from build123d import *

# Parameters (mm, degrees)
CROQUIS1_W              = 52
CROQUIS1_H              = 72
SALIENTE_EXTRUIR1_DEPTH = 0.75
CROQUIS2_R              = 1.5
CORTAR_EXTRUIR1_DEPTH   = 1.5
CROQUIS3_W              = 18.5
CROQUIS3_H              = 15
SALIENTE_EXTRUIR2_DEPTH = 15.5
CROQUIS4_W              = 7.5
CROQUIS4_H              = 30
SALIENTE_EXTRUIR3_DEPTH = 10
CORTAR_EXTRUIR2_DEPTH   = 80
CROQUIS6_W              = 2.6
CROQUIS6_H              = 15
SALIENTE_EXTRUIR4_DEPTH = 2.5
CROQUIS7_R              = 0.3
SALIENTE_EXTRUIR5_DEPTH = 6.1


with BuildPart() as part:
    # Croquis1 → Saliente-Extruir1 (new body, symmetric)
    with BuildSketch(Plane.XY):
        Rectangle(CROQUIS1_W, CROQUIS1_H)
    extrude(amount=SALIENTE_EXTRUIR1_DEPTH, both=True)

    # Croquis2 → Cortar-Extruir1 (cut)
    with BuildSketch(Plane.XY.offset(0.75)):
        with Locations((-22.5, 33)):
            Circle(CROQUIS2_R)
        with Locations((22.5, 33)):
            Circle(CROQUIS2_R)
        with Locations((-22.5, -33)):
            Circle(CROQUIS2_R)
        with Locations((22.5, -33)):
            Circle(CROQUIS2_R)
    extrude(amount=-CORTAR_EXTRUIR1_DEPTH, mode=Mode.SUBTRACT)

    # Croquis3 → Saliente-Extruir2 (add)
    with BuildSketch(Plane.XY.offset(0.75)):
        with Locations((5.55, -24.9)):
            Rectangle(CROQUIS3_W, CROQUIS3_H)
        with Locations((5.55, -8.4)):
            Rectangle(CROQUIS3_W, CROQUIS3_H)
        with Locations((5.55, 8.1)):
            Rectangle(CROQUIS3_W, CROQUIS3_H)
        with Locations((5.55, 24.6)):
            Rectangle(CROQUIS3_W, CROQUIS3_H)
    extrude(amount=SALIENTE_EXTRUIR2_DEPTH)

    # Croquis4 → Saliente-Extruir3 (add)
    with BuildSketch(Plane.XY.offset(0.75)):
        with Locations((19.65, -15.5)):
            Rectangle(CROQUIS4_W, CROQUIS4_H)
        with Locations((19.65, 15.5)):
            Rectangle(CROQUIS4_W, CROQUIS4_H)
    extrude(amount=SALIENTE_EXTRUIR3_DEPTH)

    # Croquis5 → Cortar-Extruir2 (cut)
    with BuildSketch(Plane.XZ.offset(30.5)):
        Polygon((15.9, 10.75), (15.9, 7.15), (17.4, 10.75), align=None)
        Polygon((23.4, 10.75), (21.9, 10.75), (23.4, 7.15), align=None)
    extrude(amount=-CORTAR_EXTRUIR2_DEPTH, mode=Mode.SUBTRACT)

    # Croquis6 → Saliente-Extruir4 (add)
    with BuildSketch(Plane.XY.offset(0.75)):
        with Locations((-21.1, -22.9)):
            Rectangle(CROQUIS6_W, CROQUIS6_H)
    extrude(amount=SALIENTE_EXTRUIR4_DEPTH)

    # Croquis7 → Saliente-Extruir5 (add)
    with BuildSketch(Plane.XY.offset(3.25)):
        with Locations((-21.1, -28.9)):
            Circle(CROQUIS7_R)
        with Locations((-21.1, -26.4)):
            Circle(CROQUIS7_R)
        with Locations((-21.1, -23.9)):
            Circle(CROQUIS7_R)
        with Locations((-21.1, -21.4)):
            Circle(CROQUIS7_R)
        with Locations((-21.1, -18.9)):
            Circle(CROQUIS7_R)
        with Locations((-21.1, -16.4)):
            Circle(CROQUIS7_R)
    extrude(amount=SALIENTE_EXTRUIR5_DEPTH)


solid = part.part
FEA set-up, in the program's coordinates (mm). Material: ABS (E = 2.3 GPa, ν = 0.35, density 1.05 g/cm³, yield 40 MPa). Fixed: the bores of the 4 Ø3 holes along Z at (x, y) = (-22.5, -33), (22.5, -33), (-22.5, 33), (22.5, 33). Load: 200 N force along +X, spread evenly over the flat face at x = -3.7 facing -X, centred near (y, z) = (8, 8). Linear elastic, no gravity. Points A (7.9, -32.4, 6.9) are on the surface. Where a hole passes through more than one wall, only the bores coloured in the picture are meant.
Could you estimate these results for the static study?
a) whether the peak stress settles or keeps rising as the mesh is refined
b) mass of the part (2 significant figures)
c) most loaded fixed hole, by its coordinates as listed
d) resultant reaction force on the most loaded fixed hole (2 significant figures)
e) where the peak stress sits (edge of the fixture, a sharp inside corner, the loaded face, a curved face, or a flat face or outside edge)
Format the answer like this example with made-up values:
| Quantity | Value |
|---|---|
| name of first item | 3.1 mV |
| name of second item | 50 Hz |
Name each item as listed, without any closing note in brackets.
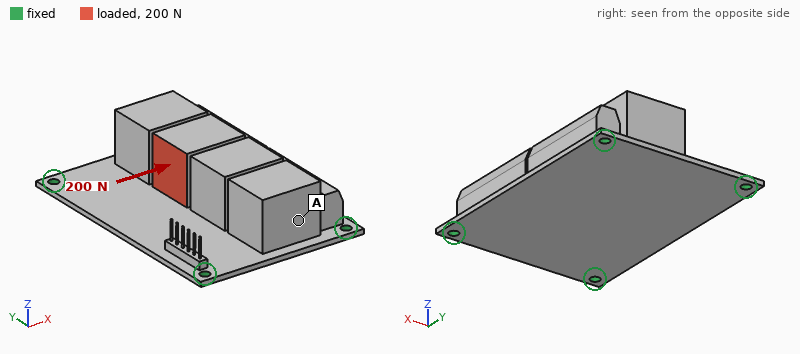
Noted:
| Quantity | Value |
|---|---|
| whether the peak stress settles or keeps rising as the mesh is refined | keeps rising |
| mass of the part | 28 g |
| most loaded fixed hole, by its coordinates as listed | (22.5, 33) |
| resultant reaction force on the most loaded fixed hole | 85 N |
| where the peak stress sits | edge of the fixture |
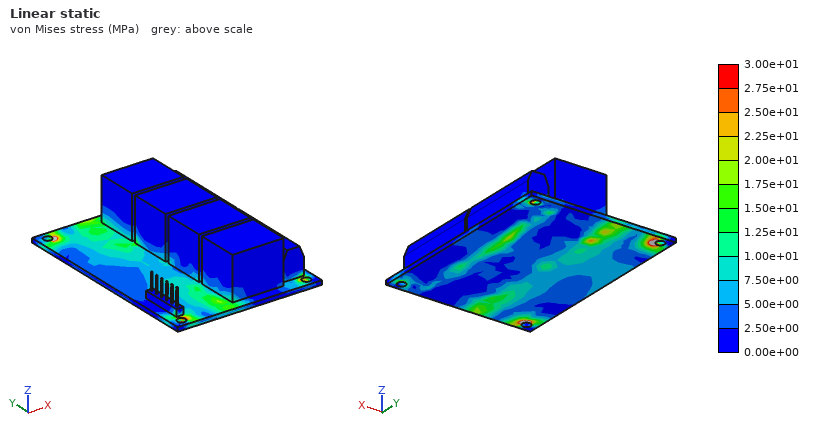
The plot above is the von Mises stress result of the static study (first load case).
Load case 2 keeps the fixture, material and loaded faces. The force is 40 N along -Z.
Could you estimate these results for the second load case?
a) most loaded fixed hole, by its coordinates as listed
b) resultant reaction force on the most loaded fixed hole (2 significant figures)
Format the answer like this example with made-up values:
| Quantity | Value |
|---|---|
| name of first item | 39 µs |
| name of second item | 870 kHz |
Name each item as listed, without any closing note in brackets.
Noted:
| Quantity | Value |
|---|---|
| most loaded fixed hole, by its coordinates as listed | (22.5, 33) |
| resultant reaction force on the most loaded fixed hole | 23 N |
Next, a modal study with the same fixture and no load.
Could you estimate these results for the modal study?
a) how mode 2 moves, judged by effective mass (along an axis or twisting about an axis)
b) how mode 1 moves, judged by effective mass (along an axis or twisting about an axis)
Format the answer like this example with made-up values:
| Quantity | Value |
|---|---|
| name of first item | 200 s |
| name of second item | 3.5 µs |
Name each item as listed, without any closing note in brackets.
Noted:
| Quantity | Value |
|---|---|
| how mode 2 moves, judged by effective mass | along X |
| how mode 1 moves, judged by effective mass | along Z |
